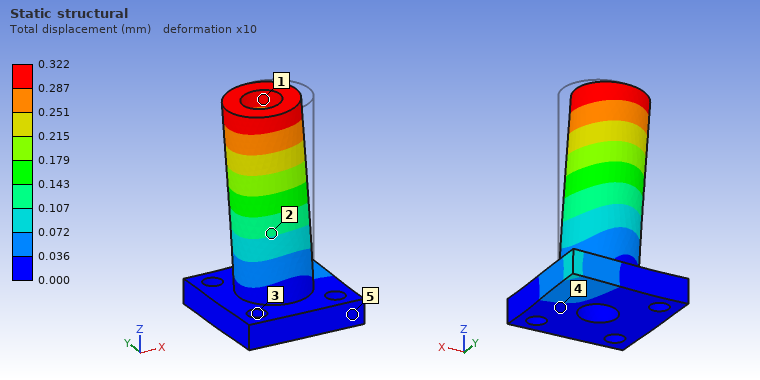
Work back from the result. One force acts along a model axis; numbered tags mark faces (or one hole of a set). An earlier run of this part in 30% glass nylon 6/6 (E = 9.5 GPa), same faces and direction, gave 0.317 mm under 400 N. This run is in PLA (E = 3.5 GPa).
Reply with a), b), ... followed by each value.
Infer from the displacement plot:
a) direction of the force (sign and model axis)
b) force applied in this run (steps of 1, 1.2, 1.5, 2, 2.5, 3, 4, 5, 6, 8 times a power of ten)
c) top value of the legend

a) -X
b) 150 N
c) 0.322 mm
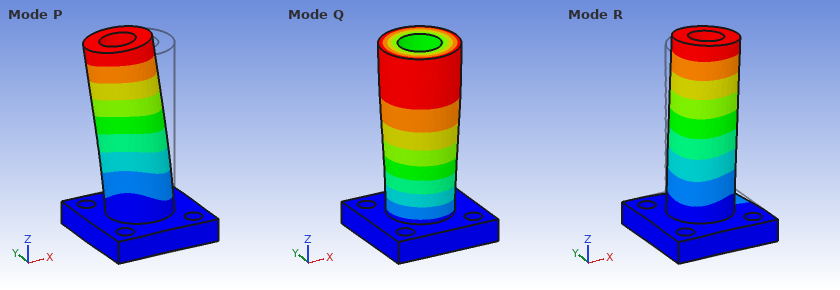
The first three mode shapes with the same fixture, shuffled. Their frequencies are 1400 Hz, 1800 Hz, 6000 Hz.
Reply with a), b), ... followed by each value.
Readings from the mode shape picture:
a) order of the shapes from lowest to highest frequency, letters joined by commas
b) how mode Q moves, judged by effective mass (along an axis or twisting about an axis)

a) R, P, Q
b) twisting about Z
